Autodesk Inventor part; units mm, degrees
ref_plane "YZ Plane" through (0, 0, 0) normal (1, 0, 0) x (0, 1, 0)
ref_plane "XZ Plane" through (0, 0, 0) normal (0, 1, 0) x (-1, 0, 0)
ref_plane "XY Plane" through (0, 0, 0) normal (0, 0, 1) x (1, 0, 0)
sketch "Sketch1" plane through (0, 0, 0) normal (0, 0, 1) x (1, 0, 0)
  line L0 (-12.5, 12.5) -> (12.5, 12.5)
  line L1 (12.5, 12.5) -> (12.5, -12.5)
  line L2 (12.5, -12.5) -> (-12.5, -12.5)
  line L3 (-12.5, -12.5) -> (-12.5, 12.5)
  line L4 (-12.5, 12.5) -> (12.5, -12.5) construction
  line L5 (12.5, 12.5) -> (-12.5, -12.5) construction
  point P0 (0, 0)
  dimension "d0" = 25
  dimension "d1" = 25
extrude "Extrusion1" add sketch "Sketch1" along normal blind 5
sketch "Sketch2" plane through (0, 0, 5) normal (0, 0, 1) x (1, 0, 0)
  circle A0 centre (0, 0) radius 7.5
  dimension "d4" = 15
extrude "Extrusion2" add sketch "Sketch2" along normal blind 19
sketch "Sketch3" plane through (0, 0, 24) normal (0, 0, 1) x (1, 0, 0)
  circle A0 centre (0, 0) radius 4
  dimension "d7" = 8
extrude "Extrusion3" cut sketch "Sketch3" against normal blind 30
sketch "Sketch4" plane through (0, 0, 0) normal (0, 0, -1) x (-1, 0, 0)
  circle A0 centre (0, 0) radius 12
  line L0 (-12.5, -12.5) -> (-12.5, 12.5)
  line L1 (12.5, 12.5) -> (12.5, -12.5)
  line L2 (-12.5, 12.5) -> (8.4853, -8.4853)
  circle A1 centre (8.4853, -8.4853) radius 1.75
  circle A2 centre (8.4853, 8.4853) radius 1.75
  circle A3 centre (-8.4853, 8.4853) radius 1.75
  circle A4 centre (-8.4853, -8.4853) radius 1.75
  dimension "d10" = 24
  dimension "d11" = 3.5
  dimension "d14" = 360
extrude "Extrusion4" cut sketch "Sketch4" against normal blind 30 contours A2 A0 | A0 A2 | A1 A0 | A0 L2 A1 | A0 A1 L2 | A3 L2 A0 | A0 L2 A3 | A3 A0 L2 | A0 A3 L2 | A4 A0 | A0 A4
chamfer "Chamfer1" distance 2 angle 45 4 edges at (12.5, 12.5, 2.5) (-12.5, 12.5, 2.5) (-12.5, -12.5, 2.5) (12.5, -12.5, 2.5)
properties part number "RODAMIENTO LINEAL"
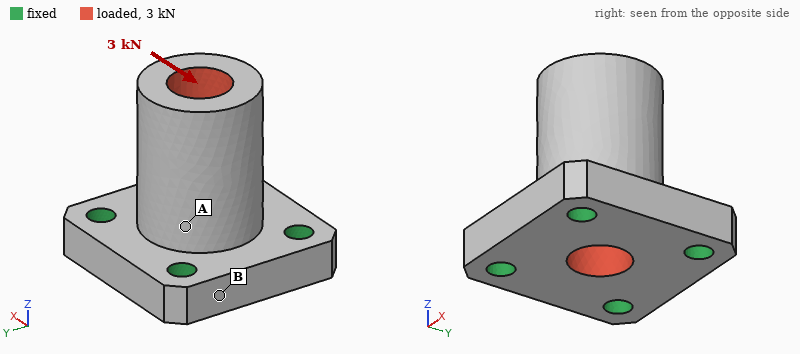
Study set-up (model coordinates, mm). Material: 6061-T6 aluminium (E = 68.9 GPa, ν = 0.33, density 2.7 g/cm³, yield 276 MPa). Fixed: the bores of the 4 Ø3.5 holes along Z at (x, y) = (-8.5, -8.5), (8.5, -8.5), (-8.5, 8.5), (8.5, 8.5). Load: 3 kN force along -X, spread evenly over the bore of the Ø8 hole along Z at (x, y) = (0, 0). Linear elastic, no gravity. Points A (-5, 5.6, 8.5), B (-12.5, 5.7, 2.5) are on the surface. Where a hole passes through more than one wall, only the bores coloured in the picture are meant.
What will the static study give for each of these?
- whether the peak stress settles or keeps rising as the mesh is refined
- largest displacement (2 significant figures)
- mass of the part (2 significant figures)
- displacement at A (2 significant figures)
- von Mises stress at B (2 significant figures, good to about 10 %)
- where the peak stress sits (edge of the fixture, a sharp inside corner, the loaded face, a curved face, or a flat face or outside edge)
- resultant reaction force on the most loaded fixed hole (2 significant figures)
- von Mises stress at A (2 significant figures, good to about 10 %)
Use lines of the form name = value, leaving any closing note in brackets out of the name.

whether the peak stress settles or keeps rising as the mesh is refined = keeps rising
largest displacement = 49 µm
mass of the part = 14 g
displacement at A = 13 µm
von Mises stress at B = 19 MPa
where the peak stress sits = edge of the fixture
resultant reaction force on the most loaded fixed hole = 1.2 kN
von Mises stress at A = 41 MPa
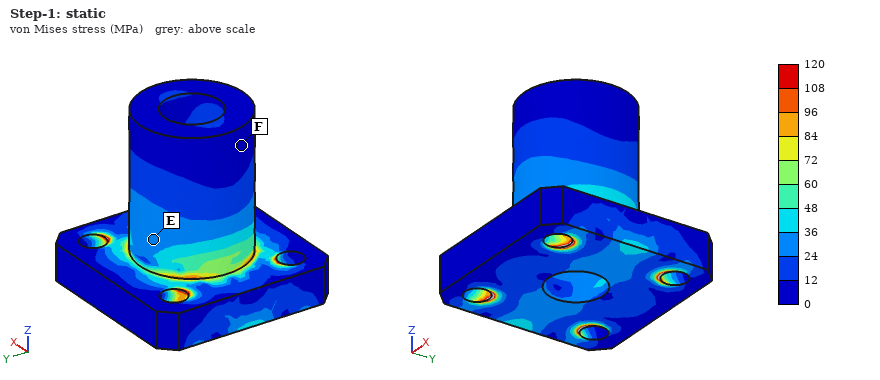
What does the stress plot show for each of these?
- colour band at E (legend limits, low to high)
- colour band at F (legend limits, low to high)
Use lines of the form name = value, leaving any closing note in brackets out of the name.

colour band at E = 24 to 36 MPa
colour band at F = 0 to 12 MPa
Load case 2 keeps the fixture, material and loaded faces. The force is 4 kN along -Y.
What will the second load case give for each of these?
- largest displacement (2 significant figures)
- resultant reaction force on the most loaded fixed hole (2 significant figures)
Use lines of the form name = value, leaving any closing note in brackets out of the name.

largest displacement = 65 µm
resultant reaction force on the most loaded fixed hole = 1.6 kN
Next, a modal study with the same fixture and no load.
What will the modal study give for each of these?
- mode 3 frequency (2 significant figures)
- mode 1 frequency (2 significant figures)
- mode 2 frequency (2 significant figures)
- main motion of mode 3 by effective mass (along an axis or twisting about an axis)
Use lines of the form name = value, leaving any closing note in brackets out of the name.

mode 3 frequency = 35 kHz
mode 1 frequency = 16 kHz
mode 2 frequency = 16 kHz
main motion of mode 3 by effective mass = along Z
